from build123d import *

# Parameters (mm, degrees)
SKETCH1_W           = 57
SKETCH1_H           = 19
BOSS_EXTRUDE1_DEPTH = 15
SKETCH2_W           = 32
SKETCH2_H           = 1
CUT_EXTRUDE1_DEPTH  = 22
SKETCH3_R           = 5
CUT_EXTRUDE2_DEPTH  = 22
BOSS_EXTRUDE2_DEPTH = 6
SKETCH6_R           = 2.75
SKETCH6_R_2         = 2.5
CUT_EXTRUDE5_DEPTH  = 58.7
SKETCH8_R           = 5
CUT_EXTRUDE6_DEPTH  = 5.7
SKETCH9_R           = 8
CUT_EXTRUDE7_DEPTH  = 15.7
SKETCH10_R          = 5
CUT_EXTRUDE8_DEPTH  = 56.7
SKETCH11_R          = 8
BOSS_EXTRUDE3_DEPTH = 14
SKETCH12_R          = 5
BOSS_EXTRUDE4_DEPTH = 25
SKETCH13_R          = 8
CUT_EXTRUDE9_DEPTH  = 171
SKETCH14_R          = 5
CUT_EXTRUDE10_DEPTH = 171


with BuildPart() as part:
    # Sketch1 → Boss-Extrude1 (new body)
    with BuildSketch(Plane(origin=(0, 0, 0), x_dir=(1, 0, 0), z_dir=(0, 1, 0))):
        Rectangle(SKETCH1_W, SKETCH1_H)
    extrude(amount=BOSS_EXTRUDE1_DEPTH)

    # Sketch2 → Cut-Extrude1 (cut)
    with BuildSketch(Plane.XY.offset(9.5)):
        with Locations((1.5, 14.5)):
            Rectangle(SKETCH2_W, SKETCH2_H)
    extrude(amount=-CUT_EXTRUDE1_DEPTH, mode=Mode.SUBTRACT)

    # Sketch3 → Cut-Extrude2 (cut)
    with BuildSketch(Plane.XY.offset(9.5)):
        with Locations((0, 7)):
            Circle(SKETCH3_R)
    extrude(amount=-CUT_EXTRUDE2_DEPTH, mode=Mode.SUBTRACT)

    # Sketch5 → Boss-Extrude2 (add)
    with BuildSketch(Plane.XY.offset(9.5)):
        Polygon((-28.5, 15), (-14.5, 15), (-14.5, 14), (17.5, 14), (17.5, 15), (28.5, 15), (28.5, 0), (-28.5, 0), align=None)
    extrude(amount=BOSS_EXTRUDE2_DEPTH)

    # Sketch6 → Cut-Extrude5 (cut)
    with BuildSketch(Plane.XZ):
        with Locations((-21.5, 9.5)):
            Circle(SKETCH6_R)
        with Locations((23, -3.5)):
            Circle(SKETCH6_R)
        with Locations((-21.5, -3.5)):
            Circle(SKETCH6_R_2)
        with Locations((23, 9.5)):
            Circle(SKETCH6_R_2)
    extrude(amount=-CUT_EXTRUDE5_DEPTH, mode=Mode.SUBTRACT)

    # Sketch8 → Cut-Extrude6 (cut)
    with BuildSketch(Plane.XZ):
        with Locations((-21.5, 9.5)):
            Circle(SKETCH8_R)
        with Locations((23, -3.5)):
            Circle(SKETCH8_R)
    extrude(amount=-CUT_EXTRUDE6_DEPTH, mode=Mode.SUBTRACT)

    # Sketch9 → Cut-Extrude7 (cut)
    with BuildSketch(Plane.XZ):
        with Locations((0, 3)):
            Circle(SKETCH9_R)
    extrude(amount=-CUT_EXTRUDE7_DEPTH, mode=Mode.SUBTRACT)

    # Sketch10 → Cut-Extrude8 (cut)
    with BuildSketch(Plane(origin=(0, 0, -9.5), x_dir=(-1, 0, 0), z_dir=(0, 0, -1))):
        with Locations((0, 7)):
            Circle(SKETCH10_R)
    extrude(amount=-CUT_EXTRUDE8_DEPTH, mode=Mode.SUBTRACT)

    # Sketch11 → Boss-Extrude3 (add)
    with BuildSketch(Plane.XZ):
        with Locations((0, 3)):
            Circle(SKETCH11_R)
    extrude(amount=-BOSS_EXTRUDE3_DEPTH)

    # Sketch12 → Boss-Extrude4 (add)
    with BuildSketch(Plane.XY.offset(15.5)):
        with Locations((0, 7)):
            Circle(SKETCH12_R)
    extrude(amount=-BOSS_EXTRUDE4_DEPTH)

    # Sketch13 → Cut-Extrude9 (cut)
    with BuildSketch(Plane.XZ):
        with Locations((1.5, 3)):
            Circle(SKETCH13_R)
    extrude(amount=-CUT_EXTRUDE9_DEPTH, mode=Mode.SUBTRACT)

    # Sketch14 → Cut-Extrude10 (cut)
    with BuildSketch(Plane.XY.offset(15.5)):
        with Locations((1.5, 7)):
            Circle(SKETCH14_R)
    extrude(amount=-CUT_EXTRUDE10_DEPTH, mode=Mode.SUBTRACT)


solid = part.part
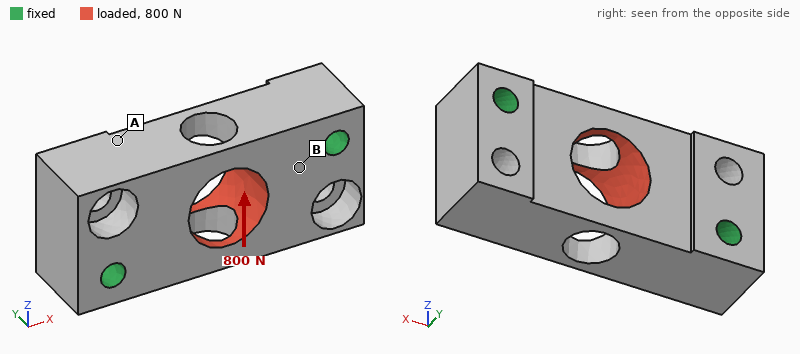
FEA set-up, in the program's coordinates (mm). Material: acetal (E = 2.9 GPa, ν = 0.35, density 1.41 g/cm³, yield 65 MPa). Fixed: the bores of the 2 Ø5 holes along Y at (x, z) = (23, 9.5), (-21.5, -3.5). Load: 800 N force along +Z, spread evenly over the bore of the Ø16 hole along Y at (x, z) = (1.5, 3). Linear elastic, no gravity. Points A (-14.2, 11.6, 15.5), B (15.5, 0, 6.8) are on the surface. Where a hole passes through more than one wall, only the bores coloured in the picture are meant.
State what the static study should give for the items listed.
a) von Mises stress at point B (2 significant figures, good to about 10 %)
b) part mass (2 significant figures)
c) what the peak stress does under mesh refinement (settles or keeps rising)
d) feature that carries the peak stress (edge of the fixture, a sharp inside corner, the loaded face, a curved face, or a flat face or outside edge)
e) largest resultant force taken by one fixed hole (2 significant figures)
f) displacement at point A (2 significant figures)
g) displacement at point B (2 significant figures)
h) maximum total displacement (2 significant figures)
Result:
4.0 MPa
21 g
keeps rising
a sharp inside corner
410 N
52 µm
26 µm
76 µm
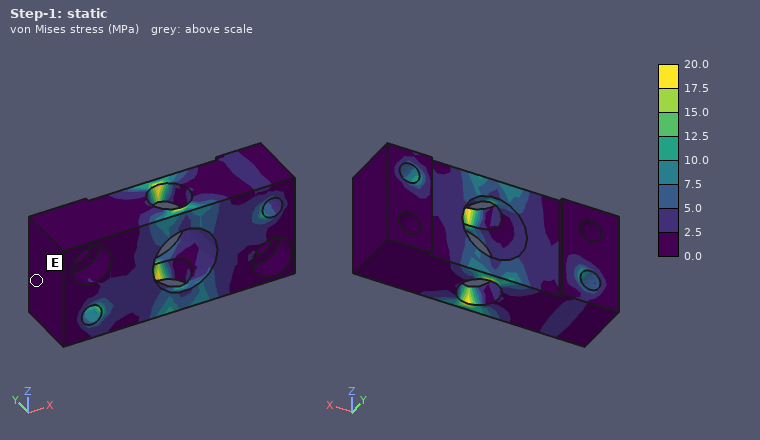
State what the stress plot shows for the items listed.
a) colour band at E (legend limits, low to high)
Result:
0.0 to 2.5 MPa
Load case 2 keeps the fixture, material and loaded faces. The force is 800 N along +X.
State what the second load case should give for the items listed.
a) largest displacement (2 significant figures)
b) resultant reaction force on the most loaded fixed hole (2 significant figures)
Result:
30 µm
400 N
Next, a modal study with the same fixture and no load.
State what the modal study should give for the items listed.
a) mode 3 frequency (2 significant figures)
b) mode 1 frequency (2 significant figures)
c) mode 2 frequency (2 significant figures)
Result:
5800 Hz
5500 Hz
5600 Hz
